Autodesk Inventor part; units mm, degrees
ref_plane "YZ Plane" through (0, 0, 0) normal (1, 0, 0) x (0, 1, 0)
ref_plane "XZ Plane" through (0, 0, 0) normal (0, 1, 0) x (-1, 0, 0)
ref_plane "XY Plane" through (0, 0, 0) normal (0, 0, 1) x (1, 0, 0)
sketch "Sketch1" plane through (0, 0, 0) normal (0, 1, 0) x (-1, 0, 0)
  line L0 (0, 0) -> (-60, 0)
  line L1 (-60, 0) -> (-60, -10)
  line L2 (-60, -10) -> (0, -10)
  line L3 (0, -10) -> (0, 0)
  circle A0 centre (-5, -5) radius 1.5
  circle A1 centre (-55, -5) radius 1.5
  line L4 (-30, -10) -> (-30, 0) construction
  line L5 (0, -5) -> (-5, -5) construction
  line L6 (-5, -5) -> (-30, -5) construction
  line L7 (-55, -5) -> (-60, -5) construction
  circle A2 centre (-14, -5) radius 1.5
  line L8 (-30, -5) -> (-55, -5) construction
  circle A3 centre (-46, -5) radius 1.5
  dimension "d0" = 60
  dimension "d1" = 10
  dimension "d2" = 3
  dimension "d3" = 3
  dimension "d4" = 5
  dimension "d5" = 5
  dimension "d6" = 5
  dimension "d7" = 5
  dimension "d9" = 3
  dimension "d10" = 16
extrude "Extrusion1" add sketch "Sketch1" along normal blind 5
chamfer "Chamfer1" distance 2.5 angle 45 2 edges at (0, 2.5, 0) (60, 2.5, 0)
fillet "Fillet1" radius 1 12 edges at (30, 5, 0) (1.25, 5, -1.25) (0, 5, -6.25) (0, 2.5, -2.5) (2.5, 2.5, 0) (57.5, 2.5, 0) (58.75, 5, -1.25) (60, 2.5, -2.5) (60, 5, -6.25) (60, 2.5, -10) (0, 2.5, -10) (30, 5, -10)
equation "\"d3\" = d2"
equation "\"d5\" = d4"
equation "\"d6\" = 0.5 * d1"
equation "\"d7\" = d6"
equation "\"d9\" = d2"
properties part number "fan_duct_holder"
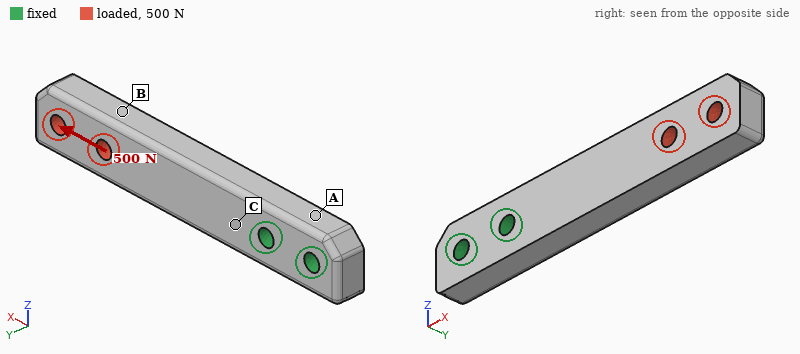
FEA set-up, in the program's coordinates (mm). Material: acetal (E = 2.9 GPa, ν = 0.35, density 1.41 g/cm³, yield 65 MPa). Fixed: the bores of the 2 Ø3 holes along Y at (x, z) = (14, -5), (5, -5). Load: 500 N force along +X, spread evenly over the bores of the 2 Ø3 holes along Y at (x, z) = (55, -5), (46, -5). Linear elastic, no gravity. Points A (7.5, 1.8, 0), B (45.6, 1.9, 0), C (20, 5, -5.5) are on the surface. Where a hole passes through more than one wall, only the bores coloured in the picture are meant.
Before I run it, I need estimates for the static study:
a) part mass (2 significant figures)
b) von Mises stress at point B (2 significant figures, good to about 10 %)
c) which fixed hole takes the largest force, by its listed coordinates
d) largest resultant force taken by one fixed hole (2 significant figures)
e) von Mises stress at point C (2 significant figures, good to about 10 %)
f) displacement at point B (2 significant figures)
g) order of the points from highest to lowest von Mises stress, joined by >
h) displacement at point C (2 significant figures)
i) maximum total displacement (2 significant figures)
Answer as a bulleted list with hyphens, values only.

- 3.9 g
- 7.3 MPa
- (14, -5)
- 440 N
- 12 MPa
- 0.11 mm
- C > B > A
- 0.023 mm
- 0.15 mm
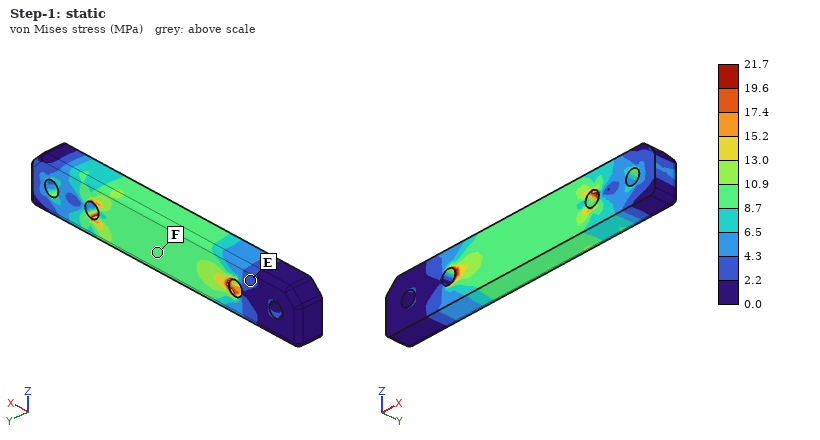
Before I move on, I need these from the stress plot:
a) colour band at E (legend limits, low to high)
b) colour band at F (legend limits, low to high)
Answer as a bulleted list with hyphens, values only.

- 2.2 to 4.3 MPa
- 8.7 to 10.9 MPa
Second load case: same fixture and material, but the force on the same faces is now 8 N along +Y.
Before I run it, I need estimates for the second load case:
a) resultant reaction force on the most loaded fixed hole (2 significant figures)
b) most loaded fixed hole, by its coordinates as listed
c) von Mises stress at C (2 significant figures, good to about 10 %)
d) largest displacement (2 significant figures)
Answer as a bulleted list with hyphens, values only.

- 14 N
- (14, -5)
- 6.1 MPa
- 0.61 mm
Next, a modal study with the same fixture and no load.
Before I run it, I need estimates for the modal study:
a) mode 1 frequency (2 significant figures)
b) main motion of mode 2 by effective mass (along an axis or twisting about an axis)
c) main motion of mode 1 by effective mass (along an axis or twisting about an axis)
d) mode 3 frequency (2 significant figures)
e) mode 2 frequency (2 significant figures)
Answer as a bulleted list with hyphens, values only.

- 580 Hz
- along Z
- along Y
- 3300 Hz
- 990 Hz
